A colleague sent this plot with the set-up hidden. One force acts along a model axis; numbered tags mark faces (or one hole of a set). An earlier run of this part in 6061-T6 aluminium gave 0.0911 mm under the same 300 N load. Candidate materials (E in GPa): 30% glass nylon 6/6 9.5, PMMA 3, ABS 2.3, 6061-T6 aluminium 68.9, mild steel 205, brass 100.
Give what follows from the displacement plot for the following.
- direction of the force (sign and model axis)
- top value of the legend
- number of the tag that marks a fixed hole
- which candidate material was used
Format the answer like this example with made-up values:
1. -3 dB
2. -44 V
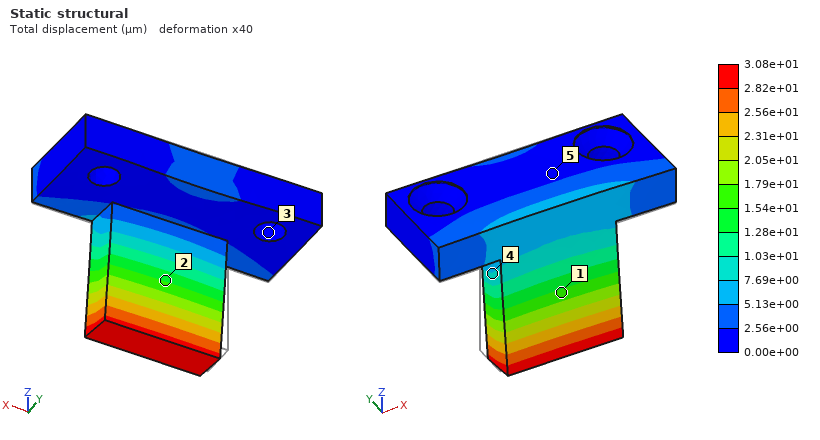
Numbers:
1. -Y
2. 3.08e+01 µm
3. 3
4. mild steel
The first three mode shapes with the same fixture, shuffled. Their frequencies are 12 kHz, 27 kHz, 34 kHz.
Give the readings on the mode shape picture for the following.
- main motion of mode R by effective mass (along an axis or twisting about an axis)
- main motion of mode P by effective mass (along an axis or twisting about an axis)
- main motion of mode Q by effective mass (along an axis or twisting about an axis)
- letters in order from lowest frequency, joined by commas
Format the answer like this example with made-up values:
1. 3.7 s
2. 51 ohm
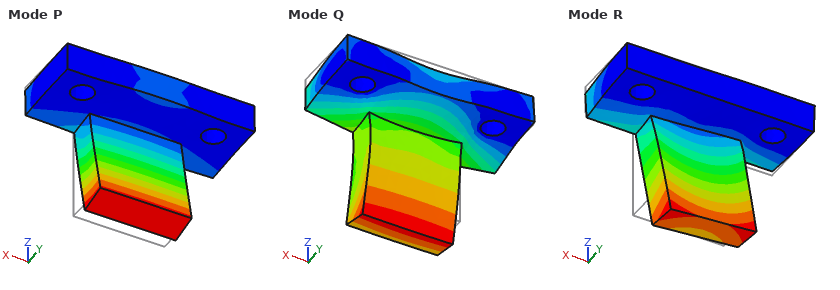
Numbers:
1. along X
2. along Y
3. along Z
4. P, R, Q
